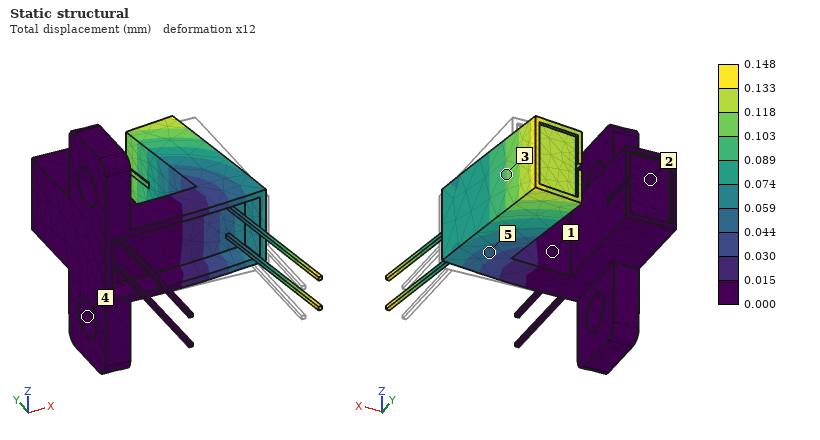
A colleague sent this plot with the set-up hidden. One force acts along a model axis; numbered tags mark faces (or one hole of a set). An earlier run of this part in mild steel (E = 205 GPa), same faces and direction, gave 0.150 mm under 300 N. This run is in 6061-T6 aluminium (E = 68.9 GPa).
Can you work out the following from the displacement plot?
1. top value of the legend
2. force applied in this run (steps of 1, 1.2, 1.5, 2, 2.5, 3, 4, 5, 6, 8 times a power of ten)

0.148 mm
100 N
